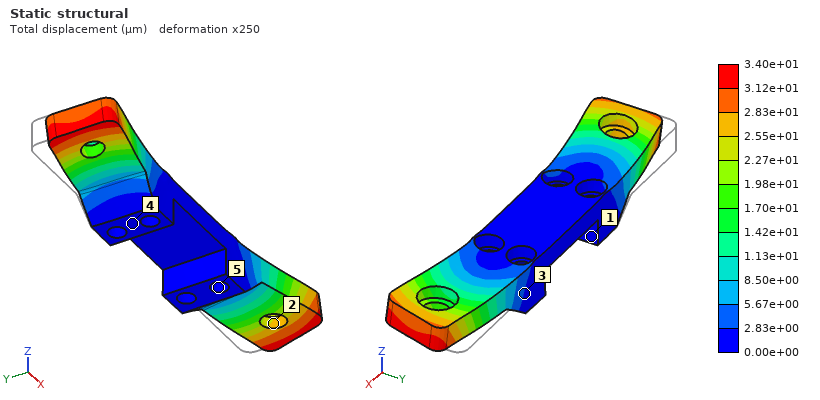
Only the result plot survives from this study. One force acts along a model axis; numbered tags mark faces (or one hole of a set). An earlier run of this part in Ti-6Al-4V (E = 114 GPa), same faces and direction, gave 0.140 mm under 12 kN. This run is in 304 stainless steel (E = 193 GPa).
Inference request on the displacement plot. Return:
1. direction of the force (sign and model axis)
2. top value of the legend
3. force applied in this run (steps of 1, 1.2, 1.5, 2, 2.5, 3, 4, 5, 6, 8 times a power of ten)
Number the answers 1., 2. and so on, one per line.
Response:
1. -Y
2. 3.40e+01 µm
3. 5 kN
